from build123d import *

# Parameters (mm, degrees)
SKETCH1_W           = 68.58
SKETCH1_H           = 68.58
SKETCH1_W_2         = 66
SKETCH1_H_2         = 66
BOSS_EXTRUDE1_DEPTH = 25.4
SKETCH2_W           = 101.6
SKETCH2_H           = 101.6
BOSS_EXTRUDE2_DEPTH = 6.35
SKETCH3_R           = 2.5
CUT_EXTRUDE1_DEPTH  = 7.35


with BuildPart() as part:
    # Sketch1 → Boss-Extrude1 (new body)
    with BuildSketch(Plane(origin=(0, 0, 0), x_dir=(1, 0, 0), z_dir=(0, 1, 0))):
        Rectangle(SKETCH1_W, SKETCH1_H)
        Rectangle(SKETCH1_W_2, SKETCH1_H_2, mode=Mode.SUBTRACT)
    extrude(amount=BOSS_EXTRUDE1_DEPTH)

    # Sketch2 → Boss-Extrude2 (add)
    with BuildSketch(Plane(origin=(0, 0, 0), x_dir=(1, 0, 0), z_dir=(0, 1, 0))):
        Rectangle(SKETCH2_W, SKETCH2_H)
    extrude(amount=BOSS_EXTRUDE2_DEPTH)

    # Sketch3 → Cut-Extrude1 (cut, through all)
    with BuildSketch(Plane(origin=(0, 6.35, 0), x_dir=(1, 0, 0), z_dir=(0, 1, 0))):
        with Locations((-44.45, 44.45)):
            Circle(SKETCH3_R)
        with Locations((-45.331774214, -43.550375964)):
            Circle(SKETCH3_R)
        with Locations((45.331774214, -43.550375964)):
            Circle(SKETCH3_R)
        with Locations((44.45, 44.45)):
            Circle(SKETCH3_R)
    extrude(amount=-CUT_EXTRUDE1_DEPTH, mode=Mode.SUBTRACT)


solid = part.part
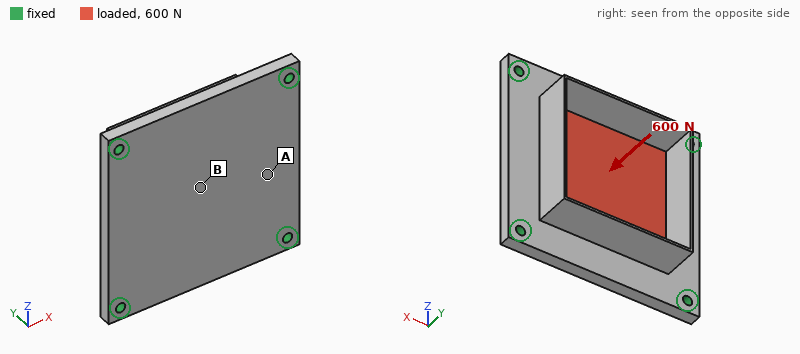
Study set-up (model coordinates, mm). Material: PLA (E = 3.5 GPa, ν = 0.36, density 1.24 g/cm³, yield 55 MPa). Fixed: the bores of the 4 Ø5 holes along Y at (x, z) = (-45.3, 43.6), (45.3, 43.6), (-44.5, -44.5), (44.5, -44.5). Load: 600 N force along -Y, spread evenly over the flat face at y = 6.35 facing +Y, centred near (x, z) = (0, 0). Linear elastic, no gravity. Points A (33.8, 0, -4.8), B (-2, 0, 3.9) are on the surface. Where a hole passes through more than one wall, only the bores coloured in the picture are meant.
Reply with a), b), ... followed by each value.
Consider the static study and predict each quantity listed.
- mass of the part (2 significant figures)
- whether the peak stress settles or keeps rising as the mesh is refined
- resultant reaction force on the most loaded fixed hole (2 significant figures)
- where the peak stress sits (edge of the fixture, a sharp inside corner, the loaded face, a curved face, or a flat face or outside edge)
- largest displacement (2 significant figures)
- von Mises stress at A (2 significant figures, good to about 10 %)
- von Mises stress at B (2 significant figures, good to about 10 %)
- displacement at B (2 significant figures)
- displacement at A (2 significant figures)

a) 89 g
b) keeps rising
c) 160 N
d) edge of the fixture
e) 0.37 mm
f) 2.4 MPa
g) 5.9 MPa
h) 0.37 mm
i) 0.21 mm
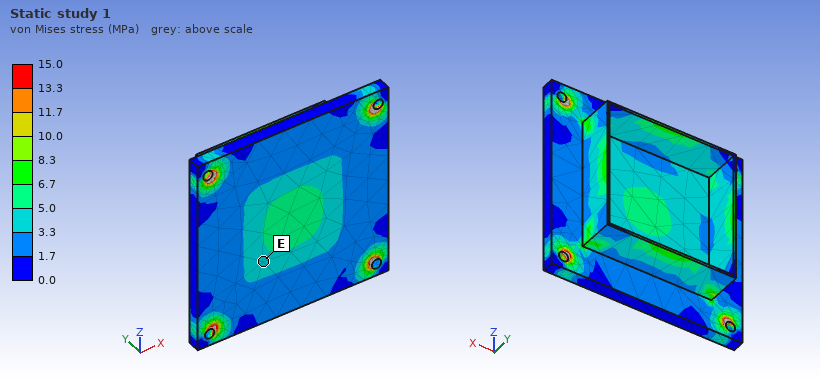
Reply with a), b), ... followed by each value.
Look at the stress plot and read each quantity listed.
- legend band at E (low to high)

a) 3.3 to 5.0 MPa
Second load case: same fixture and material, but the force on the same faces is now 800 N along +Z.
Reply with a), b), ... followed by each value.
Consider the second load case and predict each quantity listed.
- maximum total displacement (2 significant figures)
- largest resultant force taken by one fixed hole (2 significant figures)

a) 35 µm
b) 230 N
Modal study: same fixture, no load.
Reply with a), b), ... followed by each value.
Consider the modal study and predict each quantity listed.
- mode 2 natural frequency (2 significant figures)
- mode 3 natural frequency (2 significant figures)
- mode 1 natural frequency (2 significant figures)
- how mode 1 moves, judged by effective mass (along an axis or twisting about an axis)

a) 1200 Hz
b) 1300 Hz
c) 1100 Hz
d) along Y
